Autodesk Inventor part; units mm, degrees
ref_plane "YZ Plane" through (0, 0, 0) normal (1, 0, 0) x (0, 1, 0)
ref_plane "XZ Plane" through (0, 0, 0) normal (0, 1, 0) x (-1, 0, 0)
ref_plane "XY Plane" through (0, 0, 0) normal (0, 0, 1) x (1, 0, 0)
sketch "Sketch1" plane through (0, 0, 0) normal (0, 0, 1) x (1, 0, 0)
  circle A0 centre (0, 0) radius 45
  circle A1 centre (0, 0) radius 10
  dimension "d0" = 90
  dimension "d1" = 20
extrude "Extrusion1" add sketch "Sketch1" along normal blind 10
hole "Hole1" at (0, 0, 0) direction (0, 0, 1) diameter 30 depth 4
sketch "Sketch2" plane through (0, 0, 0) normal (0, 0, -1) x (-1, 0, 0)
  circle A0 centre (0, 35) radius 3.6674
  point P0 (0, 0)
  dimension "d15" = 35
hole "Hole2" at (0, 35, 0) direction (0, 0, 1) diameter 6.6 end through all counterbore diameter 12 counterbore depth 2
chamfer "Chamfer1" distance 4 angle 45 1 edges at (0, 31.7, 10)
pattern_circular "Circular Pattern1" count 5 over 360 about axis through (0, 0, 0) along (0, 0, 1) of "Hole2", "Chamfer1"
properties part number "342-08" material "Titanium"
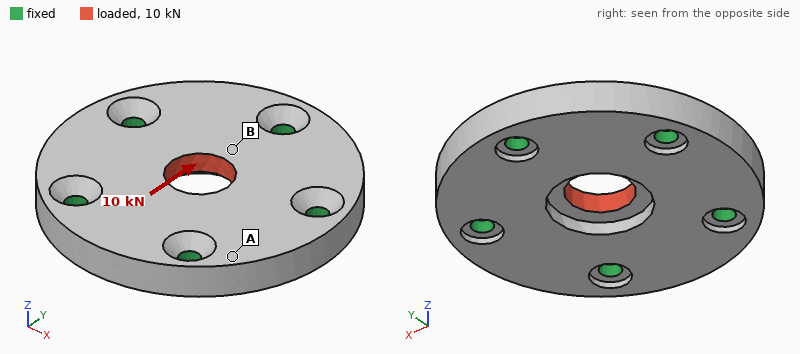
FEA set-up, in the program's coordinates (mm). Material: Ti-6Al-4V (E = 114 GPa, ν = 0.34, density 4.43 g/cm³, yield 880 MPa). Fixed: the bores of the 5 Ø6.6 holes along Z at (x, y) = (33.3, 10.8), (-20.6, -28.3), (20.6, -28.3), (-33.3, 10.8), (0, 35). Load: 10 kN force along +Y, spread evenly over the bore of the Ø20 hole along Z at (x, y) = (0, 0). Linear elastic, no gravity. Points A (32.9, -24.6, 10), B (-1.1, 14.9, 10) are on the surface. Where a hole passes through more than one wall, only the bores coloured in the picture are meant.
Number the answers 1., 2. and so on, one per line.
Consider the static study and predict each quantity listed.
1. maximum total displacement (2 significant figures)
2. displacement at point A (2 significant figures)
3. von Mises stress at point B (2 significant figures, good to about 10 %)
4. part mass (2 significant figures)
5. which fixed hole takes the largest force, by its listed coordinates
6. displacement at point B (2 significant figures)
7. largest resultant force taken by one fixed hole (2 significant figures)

1. 6.4 µm
2. 1.1 µm
3. 27 MPa
4. 240 g
5. (0, 35)
6. 4.8 µm
7. 2.7 kN
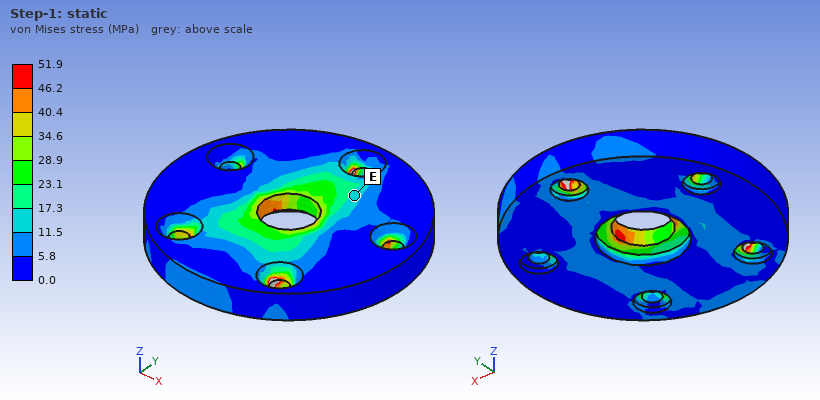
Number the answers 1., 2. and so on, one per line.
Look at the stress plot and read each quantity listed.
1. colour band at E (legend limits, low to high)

1. 11.5 to 17.3 MPa
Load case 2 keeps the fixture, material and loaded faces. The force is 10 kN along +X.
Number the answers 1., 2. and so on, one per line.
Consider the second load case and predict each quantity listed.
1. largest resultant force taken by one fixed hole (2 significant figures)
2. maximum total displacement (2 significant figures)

1. 2.6 kN
2. 6.3 µm
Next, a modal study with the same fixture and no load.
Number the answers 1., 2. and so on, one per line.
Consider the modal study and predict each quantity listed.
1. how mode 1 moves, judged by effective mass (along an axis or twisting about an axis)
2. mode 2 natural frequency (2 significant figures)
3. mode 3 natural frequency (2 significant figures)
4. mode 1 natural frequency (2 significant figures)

1. along Z
2. 13 kHz
3. 13 kHz
4. 12 kHz
